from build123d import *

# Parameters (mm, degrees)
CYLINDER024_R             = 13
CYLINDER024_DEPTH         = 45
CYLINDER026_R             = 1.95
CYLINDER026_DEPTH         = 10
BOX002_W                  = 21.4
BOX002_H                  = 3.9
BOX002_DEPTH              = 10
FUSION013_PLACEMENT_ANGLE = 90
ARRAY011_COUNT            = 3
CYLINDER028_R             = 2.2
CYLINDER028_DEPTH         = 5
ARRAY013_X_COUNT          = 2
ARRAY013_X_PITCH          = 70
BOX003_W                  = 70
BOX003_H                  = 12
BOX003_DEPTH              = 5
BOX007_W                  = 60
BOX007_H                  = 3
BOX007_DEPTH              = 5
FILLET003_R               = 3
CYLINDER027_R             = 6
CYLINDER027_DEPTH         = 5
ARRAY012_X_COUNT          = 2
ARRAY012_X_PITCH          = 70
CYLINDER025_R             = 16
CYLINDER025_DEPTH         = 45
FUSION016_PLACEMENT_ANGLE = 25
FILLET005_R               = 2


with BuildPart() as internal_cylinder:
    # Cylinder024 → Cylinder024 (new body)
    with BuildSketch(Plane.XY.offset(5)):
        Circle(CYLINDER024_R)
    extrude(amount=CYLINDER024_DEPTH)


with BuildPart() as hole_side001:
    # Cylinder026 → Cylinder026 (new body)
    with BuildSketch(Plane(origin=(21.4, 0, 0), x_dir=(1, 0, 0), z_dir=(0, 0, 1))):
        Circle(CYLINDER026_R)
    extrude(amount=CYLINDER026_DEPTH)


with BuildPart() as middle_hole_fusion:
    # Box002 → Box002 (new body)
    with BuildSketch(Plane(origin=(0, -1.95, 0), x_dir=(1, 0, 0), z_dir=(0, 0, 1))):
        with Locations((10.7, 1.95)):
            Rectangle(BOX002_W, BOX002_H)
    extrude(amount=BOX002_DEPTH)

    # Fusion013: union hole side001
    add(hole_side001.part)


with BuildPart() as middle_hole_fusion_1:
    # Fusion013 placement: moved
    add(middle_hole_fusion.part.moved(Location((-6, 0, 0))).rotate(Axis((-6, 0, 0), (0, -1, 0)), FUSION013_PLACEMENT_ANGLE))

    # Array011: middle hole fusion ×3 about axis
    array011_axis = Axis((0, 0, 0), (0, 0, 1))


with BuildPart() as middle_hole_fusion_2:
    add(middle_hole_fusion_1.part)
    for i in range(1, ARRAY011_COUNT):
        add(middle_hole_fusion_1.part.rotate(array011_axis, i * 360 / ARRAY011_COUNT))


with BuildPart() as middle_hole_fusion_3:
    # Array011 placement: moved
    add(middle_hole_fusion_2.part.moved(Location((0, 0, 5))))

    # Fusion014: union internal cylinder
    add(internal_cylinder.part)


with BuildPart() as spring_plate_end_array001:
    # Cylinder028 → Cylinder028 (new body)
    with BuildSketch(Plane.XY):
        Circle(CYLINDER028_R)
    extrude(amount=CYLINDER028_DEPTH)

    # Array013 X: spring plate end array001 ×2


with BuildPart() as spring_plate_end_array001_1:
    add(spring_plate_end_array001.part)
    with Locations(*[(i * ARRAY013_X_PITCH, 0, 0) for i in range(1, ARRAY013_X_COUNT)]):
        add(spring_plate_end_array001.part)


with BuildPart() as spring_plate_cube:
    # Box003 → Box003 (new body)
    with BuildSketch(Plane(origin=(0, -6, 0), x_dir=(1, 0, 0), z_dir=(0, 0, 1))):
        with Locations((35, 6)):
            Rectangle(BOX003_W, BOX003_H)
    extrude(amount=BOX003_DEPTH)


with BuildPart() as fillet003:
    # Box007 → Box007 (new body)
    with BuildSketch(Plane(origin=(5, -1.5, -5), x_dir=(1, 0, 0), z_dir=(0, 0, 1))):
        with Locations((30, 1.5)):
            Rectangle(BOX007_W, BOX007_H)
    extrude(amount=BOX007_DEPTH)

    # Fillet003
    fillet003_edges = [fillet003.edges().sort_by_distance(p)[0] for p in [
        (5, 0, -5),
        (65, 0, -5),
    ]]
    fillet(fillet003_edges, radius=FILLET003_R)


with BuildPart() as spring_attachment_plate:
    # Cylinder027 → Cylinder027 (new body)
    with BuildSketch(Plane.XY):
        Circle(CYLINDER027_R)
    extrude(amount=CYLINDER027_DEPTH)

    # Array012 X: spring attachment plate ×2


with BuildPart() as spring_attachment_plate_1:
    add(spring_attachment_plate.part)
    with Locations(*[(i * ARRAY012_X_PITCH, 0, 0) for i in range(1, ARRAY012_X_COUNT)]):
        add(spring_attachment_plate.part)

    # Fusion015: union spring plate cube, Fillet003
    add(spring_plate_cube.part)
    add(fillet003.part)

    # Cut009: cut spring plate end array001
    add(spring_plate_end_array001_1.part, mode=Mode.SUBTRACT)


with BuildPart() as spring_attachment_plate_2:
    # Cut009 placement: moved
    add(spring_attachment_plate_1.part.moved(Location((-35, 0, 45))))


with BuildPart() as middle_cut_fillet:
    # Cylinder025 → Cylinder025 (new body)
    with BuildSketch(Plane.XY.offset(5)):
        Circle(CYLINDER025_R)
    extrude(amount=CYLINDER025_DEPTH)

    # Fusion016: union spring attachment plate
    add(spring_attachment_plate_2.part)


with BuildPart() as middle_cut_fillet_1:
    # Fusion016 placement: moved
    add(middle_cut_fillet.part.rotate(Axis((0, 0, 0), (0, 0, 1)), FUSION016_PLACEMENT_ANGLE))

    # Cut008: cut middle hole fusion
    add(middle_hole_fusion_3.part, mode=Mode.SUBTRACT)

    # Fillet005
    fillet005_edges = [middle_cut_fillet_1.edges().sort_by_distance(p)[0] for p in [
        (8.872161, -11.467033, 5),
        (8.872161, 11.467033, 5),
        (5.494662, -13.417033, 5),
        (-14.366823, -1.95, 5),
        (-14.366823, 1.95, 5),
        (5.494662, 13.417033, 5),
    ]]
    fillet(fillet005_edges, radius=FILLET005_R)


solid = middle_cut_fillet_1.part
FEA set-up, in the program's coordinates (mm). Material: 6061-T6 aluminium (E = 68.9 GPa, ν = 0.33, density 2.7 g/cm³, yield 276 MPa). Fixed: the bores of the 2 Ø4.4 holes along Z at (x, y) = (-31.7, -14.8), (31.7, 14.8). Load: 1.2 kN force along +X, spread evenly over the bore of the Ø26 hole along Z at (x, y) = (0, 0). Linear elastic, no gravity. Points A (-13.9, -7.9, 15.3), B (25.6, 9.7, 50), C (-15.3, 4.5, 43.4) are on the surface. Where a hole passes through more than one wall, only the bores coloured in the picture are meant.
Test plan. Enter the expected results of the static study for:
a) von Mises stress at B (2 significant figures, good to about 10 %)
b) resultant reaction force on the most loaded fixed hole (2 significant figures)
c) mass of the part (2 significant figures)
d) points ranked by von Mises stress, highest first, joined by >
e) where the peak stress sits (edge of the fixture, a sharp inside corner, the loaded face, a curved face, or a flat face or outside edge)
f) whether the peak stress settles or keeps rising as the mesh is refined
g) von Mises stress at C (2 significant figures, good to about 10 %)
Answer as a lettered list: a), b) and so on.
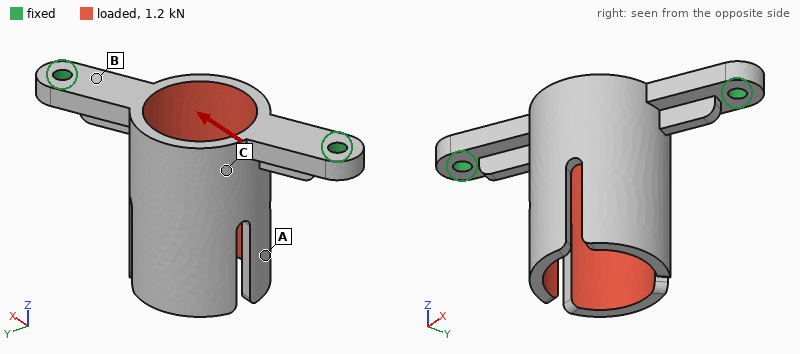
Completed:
a) 80 MPa
b) 720 N
c) 39 g
d) B > C > A
e) edge of the fixture
f) keeps rising
g) 20 MPa
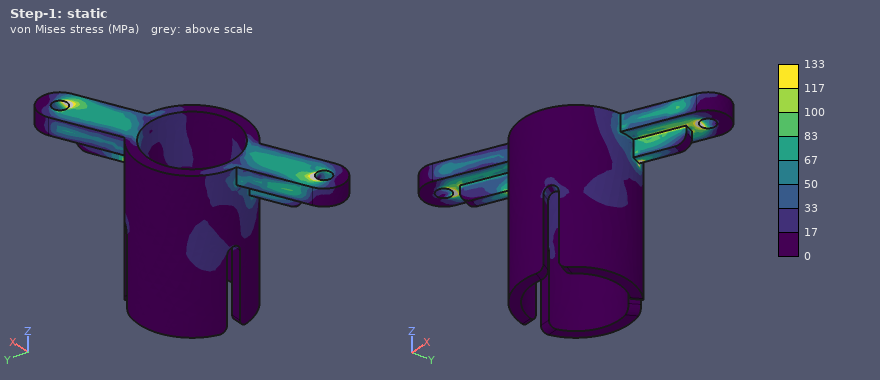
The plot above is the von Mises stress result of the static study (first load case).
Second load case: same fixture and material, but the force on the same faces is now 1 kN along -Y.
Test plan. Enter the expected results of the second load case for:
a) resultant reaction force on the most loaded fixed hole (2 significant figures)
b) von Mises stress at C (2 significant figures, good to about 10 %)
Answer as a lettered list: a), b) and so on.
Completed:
a) 530 N
b) 26 MPa
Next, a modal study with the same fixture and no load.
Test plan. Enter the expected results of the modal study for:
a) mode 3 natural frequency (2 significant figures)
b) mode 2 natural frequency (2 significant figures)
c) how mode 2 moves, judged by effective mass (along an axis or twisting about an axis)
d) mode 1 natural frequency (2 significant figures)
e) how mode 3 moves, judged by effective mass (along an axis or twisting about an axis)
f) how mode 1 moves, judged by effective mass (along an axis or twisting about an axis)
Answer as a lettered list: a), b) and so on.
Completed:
a) 3800 Hz
b) 3300 Hz
c) along Z
d) 1200 Hz
e) along X
f) along Y
